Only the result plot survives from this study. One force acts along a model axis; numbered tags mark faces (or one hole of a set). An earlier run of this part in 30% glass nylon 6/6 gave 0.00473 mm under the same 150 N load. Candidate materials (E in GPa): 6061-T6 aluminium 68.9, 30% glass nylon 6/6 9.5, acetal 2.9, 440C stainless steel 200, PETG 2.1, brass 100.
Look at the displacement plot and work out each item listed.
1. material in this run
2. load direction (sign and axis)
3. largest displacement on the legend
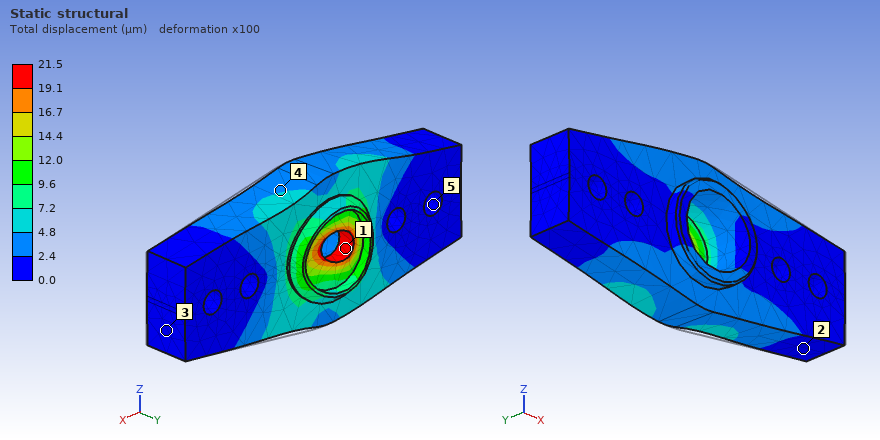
PETG
-X
21.5 µm
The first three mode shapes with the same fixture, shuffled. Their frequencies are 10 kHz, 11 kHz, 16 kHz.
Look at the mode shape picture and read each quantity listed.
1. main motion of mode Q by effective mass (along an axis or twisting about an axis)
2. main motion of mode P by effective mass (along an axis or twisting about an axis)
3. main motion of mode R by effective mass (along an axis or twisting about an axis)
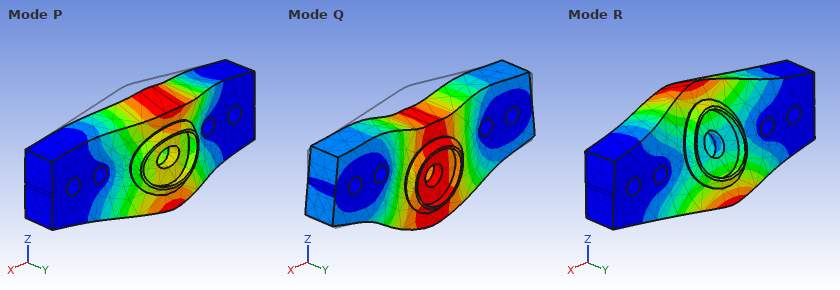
along Z
along Y
twisting about X
